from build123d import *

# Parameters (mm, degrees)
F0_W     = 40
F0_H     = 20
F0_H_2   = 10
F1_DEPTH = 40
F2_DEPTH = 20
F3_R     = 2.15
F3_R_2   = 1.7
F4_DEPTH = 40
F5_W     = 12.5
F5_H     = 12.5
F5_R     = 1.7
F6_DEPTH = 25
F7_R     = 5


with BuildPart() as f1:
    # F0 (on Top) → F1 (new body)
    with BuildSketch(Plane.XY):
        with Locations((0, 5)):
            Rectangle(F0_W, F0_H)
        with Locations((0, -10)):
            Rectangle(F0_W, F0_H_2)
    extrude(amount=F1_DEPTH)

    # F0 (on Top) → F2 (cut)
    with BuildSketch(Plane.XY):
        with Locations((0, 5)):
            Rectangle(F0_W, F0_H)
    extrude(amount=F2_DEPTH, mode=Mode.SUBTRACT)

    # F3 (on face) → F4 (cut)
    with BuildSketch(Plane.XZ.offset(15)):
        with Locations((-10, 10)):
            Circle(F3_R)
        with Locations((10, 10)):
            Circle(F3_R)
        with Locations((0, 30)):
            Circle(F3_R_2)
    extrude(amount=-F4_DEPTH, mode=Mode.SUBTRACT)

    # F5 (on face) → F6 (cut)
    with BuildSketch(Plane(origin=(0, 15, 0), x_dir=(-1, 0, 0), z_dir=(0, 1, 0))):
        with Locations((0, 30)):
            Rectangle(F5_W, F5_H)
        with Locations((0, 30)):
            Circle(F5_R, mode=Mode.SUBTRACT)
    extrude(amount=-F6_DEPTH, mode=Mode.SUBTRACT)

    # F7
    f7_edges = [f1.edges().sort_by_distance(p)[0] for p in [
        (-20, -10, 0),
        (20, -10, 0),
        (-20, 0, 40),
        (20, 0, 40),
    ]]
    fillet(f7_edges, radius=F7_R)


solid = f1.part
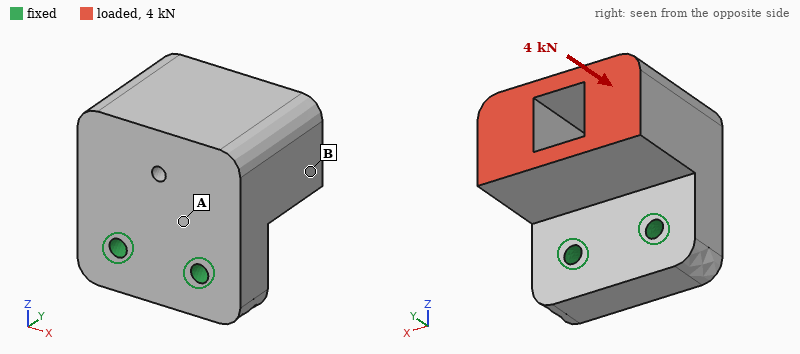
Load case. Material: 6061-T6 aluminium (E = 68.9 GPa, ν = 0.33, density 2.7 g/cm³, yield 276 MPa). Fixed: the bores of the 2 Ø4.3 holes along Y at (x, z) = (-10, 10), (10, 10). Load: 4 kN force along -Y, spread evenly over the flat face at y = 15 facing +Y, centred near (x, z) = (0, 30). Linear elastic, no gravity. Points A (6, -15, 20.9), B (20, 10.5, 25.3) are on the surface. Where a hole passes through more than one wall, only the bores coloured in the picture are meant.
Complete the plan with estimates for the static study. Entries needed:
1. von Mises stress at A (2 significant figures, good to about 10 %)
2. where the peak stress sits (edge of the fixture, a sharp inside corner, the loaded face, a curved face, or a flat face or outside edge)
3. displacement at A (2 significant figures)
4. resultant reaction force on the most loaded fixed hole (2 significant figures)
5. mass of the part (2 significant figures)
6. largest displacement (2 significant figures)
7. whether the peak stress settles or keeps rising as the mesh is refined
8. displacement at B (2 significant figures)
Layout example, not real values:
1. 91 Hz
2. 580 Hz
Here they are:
1. 47 MPa
2. edge of the fixture
3. 0.030 mm
4. 2.0 kN
5. 74 g
6. 0.14 mm
7. keeps rising
8. 0.090 mm
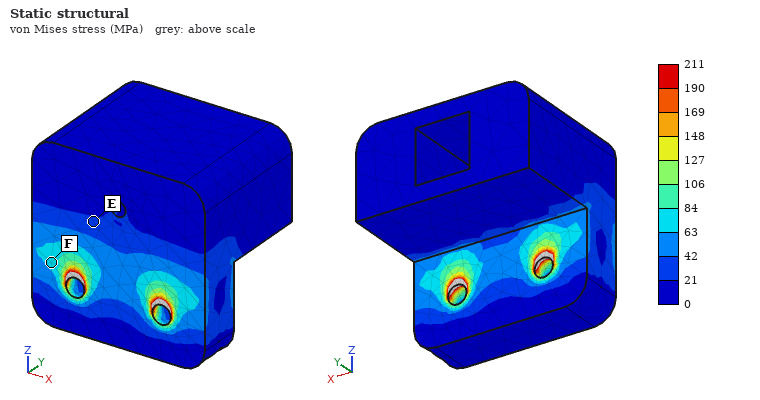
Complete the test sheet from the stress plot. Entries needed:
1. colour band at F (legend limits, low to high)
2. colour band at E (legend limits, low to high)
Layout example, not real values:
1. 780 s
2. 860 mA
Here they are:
1. 63 to 84 MPa
2. 21 to 42 MPa
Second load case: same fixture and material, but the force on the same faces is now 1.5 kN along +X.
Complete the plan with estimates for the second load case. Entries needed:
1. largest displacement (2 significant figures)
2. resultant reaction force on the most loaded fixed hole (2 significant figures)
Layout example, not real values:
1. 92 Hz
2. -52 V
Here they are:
1. 38 µm
2. 2.0 kN
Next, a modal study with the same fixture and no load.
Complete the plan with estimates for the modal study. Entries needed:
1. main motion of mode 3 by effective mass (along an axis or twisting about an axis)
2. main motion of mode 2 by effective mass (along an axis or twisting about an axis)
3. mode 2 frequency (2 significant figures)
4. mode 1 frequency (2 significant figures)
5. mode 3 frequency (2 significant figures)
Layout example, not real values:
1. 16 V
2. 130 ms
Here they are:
1. along X
2. along X
3. 7200 Hz
4. 4000 Hz
5. 11 kHz
